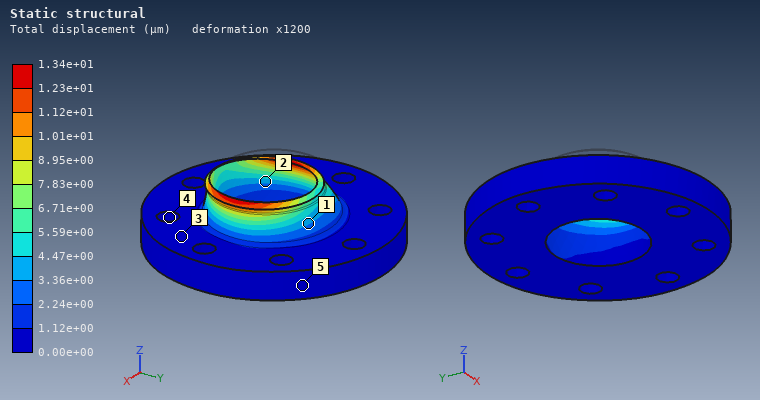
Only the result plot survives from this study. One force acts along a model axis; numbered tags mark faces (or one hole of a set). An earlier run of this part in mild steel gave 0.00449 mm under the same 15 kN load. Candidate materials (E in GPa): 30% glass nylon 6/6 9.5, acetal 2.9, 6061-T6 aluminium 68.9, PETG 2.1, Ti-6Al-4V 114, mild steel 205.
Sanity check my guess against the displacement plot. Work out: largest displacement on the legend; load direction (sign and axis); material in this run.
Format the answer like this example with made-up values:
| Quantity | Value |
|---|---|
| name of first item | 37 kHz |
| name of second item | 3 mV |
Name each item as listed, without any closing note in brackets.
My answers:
| Quantity | Value |
|---|---|
| largest displacement on the legend | 1.34e+01 µm |
| load direction | +X |
| material in this run | 6061-T6 aluminium |
